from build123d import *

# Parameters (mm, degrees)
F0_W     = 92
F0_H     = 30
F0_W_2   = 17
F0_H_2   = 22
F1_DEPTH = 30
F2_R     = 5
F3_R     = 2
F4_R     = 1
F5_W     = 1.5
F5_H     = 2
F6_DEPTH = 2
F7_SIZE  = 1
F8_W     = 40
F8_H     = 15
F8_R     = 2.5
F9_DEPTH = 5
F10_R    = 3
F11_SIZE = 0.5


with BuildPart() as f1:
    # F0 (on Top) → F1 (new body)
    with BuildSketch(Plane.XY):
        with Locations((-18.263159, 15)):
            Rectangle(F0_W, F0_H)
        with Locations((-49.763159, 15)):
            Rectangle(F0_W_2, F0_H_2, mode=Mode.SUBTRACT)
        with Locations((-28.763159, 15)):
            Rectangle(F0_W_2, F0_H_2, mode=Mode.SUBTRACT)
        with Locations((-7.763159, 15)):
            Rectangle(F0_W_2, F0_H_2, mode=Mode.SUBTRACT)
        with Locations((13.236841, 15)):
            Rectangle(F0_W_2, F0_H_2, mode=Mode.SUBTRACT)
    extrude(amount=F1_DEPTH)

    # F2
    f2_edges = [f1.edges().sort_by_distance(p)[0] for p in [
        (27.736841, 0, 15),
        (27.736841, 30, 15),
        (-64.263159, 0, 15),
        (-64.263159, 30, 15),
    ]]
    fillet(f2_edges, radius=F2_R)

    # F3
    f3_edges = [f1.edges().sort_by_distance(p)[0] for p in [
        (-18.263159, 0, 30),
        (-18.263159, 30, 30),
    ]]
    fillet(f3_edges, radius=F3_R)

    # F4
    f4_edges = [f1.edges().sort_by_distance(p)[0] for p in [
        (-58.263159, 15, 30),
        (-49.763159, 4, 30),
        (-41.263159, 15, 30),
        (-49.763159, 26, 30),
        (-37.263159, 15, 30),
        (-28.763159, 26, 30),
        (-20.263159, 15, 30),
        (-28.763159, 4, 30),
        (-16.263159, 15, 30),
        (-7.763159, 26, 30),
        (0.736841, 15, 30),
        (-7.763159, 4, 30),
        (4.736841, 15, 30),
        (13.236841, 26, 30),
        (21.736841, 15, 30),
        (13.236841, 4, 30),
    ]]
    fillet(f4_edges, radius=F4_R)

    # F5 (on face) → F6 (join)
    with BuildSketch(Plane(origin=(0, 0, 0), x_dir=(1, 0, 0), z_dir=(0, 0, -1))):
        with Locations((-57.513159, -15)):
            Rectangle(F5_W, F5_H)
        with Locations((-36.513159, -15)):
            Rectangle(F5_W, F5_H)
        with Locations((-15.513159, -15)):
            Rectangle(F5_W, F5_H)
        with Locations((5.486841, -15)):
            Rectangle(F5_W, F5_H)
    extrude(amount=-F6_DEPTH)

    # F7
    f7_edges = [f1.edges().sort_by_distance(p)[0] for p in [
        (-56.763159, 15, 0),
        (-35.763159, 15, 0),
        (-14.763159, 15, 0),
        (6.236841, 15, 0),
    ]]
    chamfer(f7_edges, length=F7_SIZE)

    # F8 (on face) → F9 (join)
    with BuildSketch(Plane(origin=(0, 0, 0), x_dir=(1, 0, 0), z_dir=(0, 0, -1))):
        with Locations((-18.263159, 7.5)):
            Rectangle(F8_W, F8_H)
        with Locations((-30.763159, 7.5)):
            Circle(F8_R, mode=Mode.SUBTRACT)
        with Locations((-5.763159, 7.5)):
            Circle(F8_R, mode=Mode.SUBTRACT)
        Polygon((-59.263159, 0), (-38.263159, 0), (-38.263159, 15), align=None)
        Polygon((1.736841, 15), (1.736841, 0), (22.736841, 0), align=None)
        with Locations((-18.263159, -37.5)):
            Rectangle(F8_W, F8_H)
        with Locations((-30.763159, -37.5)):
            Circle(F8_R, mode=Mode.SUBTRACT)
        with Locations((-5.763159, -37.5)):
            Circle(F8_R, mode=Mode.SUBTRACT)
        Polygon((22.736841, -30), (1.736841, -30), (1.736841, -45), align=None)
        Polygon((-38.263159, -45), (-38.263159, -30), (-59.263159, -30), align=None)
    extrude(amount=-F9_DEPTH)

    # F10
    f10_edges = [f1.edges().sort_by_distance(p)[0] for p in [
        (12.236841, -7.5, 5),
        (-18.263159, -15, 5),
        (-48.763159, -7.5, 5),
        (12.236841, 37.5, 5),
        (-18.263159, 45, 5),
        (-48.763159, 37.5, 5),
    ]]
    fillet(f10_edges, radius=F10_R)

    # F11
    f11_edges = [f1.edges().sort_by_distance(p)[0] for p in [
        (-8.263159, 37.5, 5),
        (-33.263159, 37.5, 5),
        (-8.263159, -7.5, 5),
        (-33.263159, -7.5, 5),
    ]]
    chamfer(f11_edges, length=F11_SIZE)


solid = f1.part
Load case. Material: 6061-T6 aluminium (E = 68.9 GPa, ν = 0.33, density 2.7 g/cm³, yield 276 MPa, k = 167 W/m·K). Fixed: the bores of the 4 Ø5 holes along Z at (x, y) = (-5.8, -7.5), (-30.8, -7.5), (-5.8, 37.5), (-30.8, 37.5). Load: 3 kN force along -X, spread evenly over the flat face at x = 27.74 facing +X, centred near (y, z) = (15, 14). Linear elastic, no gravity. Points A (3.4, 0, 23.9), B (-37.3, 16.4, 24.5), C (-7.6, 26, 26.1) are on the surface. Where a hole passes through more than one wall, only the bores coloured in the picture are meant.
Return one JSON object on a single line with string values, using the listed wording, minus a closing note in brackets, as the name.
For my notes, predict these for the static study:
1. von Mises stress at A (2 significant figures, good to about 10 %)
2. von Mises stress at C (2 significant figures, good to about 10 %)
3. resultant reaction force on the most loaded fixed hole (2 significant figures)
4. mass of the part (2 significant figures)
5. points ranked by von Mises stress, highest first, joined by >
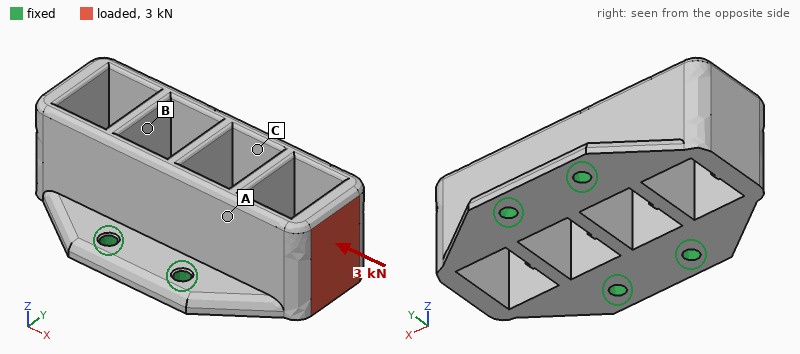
{"von Mises stress at A": "21 MPa", "von Mises stress at C": "11 MPa", "resultant reaction force on the most loaded fixed hole": "1.1 kN", "mass of the part": "120 g", "points ranked by von Mises stress, highest first, joined by >": "A > C > B"}
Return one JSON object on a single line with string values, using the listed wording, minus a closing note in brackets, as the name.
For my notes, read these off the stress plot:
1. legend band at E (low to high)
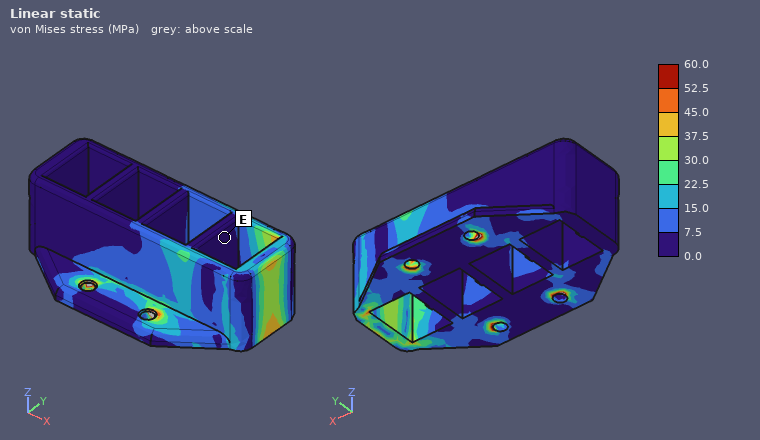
{"legend band at E": "0.0 to 7.5 MPa"}
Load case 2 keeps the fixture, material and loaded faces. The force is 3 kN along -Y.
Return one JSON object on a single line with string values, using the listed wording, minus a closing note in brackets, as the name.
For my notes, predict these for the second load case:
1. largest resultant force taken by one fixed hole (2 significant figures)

{"largest resultant force taken by one fixed hole": "2.7 kN"}
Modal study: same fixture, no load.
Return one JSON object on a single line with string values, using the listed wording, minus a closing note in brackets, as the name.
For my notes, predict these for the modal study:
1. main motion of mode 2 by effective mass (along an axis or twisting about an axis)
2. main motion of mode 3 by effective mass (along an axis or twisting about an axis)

{"main motion of mode 2 by effective mass": "twisting about Z", "main motion of mode 3 by effective mass": "along Y"}
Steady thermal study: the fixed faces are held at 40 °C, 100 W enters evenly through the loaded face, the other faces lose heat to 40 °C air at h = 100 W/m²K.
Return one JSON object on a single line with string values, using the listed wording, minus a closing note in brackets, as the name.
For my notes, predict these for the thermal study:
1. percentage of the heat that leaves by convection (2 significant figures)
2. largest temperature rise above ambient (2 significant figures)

{"percentage of the heat that leaves by convection": "32 %", "largest temperature rise above ambient": "73 K"}
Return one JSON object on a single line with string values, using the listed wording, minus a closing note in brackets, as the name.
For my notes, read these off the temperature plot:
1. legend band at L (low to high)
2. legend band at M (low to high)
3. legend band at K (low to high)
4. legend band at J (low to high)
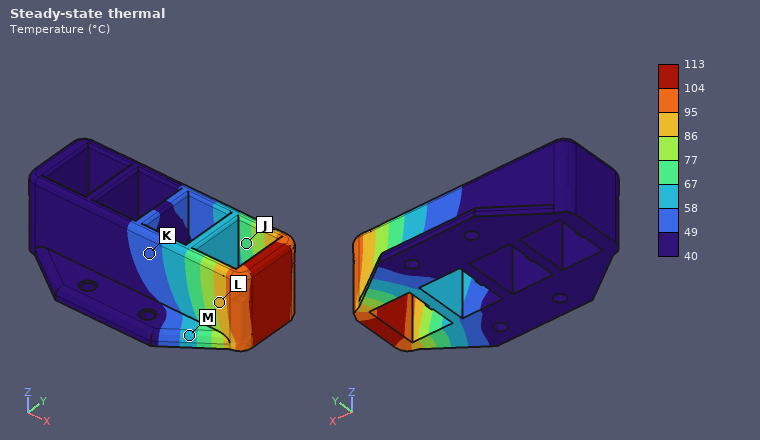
{"legend band at L": "86 to 95 °C", "legend band at M": "58 to 67 °C", "legend band at K": "49 to 58 °C", "legend band at J": "67 to 77 °C"}
